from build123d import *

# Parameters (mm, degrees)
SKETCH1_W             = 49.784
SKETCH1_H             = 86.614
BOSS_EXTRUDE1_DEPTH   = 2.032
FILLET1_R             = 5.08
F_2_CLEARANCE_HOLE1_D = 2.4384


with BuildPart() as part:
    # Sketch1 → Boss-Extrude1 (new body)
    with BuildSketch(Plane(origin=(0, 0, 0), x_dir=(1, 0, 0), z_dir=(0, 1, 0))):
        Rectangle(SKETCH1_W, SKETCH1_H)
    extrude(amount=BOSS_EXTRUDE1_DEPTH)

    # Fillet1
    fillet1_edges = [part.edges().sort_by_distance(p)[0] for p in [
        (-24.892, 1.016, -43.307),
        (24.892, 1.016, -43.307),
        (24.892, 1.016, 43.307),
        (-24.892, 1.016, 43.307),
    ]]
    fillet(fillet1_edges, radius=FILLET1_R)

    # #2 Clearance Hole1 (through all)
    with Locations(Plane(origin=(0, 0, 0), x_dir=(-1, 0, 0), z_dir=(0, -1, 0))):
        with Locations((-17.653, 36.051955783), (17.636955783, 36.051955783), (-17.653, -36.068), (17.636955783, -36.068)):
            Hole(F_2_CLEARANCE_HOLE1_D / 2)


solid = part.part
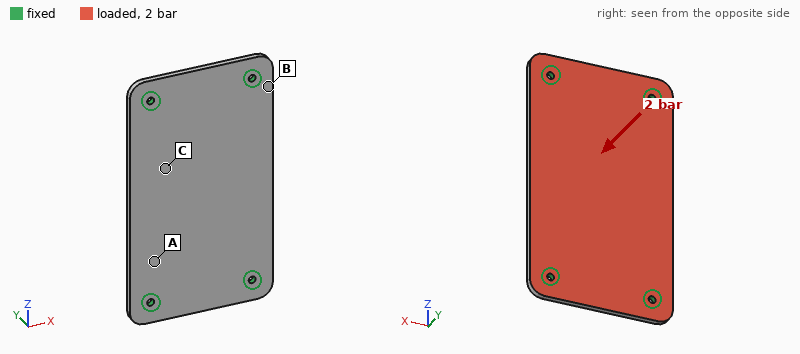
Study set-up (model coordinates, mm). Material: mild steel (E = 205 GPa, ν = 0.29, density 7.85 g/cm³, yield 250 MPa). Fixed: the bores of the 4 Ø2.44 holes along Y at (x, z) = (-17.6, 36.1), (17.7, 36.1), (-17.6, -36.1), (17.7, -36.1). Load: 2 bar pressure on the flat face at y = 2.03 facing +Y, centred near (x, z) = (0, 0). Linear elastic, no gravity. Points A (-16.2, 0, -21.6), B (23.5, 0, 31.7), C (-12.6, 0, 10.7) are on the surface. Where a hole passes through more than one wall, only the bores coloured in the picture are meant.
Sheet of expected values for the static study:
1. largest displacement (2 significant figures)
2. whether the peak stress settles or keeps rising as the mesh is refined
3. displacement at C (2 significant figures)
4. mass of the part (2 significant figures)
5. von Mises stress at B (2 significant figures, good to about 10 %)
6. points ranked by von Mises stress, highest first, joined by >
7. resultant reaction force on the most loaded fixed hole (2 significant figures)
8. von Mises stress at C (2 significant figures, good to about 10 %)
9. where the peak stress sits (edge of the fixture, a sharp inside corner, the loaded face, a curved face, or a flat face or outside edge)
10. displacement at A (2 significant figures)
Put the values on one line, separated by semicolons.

0.12 mm; keeps rising; 0.10 mm; 68 g; 96 MPa; B > C > A; 210 N; 50 MPa; edge of the fixture; 0.054 mm
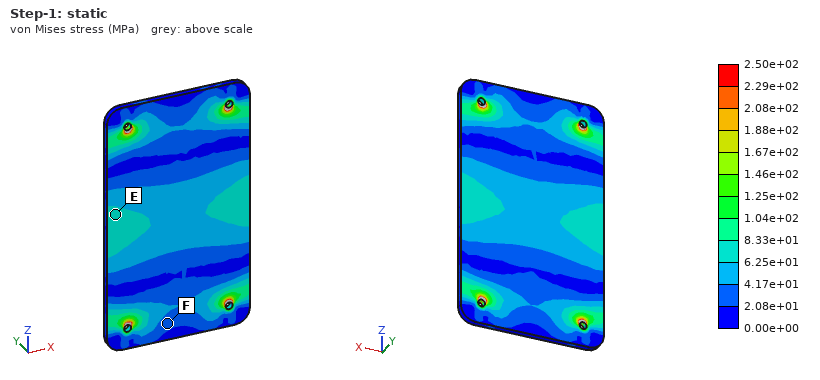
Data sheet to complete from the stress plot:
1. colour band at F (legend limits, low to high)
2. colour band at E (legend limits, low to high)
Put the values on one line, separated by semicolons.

2.08e+01 to 4.17e+01 MPa; 6.25e+01 to 8.33e+01 MPa
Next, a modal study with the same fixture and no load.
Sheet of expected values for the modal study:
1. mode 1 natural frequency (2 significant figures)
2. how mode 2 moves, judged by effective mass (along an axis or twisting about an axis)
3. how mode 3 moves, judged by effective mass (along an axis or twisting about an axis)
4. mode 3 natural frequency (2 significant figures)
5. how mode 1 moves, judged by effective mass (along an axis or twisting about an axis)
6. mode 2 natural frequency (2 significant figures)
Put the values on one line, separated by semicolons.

1800 Hz; twisting about Z; twisting about X; 5000 Hz; along Y; 2800 Hz
